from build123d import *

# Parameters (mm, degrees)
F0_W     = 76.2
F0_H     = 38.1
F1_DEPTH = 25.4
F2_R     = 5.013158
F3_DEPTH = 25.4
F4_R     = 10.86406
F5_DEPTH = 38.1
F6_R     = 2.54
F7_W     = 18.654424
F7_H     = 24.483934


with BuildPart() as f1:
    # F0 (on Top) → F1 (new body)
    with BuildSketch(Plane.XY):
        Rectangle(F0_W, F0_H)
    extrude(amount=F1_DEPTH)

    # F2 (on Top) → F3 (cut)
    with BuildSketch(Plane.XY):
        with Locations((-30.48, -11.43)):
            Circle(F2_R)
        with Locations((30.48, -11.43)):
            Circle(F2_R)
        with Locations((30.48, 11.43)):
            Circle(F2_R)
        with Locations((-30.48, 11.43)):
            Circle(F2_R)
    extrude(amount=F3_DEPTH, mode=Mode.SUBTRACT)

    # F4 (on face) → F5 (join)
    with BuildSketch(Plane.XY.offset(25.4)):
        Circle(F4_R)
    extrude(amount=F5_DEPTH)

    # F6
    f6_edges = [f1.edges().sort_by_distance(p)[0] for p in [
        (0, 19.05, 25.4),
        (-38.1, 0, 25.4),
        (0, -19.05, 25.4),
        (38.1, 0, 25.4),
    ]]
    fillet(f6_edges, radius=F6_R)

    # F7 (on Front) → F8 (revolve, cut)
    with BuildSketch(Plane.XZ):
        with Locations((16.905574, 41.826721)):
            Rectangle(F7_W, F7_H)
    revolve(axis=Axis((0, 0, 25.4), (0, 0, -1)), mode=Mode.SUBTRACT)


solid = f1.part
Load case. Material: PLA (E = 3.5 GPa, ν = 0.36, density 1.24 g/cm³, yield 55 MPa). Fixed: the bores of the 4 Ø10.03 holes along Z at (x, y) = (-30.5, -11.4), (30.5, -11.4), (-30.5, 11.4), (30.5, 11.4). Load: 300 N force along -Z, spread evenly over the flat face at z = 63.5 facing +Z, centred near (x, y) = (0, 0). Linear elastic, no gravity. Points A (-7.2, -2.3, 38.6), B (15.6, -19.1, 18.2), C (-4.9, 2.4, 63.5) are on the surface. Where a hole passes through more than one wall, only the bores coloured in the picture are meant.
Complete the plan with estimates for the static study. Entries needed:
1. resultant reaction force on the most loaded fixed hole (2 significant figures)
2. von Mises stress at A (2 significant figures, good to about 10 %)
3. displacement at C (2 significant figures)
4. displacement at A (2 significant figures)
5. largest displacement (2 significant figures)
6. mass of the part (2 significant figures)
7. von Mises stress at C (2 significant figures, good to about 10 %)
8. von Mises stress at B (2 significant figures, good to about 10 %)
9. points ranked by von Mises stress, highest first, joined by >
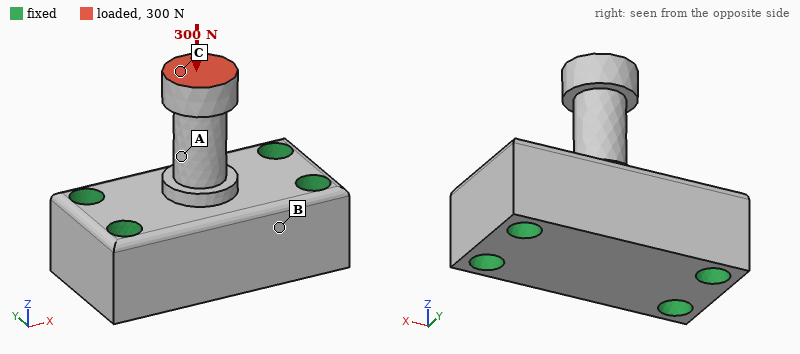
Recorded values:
78 N
1.7 MPa
21 µm
11 µm
21 µm
93 g
1.1 MPa
0.32 MPa
A > C > B
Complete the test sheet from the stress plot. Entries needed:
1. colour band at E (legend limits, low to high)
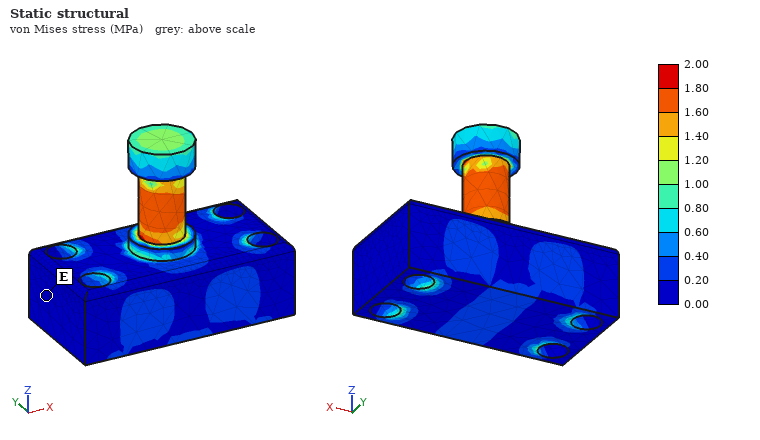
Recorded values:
0.00 to 0.20 MPa
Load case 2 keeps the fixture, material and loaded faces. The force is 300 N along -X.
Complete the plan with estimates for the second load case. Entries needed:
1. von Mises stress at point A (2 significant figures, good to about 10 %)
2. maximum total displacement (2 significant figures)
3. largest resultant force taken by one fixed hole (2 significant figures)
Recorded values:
21 MPa
0.68 mm
180 N
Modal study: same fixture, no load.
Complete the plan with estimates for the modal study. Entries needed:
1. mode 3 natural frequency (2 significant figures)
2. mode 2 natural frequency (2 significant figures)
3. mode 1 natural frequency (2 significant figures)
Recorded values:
4300 Hz
1800 Hz
1700 Hz
